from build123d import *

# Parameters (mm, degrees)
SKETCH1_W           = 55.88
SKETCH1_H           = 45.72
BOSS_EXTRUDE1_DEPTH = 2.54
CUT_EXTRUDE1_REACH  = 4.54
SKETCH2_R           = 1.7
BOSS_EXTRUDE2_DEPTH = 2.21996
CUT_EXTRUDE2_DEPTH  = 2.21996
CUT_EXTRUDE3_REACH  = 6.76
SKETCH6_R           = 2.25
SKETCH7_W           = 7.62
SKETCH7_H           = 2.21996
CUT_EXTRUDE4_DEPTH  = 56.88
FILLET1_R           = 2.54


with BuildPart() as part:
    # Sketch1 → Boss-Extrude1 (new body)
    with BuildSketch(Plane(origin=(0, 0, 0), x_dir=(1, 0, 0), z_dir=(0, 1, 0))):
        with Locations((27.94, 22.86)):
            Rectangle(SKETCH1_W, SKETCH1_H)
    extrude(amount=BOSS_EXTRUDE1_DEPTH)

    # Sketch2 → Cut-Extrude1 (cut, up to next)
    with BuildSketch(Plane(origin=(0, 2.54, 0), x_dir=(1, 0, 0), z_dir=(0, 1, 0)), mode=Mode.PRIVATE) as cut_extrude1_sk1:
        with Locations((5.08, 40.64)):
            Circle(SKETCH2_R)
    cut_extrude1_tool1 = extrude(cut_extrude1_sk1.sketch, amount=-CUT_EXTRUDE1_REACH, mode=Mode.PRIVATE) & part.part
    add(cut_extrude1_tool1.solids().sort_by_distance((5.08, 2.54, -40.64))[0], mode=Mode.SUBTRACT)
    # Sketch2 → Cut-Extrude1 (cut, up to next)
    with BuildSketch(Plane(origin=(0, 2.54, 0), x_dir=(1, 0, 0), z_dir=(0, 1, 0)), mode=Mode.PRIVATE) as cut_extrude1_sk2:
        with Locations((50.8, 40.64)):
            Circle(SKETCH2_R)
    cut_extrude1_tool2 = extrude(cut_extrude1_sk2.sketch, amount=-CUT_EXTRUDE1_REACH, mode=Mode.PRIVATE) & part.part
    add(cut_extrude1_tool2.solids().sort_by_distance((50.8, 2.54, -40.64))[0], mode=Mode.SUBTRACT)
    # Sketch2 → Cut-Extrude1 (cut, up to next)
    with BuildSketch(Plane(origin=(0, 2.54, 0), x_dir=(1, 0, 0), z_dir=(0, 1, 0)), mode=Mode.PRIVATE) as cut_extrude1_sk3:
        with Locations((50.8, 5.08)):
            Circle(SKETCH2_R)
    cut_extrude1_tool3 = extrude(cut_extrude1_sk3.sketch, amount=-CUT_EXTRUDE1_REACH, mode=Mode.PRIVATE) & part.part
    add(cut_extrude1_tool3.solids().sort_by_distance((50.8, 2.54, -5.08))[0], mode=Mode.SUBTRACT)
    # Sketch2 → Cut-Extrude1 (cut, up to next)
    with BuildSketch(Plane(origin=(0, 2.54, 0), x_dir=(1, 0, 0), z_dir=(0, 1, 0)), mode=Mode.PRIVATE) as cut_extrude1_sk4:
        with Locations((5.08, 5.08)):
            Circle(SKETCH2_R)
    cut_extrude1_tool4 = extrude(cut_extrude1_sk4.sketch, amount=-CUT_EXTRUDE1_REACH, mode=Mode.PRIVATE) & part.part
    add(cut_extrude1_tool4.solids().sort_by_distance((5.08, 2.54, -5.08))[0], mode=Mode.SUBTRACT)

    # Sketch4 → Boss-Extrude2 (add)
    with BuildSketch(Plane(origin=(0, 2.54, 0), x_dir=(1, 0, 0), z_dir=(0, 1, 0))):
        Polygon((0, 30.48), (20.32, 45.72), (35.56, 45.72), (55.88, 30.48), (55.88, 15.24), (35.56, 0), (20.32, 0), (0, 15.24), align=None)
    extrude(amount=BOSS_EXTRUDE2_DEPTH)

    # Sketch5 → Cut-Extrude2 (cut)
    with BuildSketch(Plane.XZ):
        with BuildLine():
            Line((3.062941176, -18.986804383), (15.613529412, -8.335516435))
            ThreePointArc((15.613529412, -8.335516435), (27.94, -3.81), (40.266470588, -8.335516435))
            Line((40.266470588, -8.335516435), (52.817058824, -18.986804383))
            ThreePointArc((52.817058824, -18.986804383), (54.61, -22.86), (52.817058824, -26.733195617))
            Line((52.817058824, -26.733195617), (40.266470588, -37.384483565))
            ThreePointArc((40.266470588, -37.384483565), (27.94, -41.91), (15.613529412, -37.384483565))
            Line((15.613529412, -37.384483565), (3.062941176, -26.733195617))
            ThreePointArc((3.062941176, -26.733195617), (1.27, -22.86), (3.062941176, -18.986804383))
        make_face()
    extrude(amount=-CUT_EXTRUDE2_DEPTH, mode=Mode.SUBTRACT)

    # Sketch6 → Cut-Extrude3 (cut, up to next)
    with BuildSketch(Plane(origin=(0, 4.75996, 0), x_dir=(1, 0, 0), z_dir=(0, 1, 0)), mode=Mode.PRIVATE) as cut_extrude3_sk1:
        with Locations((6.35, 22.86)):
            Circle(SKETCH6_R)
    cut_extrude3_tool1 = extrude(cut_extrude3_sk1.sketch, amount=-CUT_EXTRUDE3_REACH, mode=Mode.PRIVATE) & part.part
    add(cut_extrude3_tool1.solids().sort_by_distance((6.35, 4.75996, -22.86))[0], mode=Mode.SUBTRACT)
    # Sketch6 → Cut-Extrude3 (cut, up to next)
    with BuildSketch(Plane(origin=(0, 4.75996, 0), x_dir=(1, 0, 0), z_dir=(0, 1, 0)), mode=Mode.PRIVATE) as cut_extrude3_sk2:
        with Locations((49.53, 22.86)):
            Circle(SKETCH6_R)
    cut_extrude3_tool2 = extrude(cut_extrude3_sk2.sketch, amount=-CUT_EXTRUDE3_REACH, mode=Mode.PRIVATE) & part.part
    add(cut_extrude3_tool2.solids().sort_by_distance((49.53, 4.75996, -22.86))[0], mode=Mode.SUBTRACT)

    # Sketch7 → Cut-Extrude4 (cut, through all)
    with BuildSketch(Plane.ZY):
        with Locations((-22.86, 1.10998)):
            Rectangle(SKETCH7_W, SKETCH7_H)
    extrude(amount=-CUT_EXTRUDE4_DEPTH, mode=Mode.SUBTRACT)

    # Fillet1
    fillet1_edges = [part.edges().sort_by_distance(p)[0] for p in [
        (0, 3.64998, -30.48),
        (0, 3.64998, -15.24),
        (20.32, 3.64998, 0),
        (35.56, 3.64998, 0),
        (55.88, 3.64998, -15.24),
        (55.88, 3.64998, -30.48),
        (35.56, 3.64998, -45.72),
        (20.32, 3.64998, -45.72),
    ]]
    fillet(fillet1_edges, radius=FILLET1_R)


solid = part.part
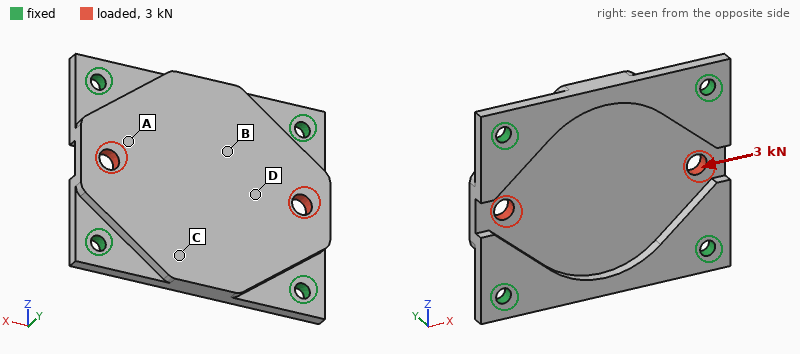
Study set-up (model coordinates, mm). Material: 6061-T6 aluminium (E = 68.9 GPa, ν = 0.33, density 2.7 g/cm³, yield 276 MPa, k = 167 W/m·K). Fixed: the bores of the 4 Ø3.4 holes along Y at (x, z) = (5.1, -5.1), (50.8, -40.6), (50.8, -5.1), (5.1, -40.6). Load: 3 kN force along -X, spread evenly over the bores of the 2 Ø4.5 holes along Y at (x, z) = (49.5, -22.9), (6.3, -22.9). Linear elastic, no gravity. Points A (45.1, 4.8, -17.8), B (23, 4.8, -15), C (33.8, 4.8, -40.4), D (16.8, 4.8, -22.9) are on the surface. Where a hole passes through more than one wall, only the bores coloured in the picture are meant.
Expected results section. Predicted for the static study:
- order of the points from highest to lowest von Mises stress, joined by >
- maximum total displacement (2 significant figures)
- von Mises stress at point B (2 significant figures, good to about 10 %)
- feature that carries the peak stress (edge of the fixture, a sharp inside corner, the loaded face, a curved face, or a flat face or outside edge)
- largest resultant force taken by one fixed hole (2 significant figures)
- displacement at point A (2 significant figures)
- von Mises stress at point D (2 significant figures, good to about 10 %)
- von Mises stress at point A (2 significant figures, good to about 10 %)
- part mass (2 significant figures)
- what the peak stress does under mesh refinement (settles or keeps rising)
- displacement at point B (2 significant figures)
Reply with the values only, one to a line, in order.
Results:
A > D > B > C
18 µm
16 MPa
edge of the fixture
770 N
12 µm
27 MPa
34 MPa
20 g
keeps rising
7.6 µm
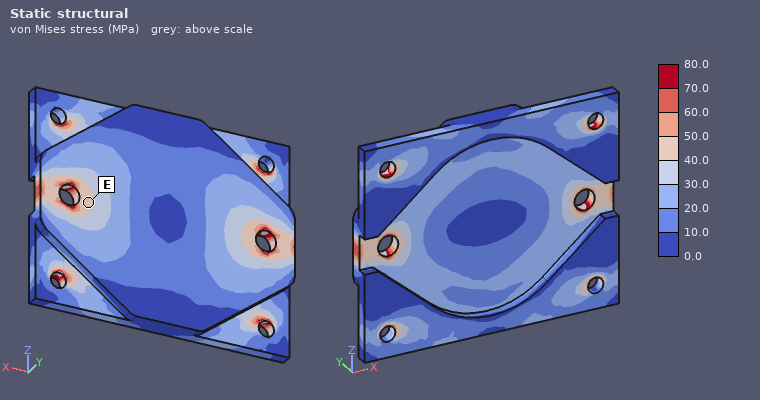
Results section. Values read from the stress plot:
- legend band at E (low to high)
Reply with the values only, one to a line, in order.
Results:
40.0 to 50.0 MPa
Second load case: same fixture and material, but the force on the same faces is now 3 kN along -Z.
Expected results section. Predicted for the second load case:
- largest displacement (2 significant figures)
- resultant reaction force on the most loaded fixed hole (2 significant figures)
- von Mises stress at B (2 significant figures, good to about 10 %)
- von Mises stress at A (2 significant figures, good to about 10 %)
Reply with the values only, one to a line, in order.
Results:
9.1 µm
760 N
6.7 MPa
13 MPa
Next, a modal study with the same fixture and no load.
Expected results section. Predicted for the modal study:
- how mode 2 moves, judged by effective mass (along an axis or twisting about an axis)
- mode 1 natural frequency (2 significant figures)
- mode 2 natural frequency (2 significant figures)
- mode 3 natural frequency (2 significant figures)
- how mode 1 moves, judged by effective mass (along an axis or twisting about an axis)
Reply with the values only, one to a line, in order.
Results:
twisting about X
7400 Hz
9500 Hz
12 kHz
along Y
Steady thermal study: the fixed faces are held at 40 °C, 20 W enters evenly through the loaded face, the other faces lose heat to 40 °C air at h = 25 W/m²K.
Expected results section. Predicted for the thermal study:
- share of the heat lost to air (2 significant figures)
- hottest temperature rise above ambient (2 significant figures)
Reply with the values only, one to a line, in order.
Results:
3.9 %
13 K
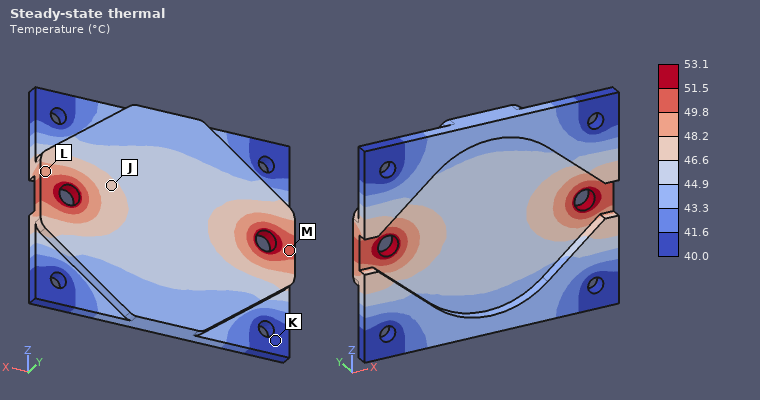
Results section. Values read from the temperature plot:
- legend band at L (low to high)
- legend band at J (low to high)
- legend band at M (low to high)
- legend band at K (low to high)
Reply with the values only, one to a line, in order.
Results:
48.2 to 49.8 °C
46.6 to 48.2 °C
49.8 to 51.5 °C
40.0 to 41.6 °C
